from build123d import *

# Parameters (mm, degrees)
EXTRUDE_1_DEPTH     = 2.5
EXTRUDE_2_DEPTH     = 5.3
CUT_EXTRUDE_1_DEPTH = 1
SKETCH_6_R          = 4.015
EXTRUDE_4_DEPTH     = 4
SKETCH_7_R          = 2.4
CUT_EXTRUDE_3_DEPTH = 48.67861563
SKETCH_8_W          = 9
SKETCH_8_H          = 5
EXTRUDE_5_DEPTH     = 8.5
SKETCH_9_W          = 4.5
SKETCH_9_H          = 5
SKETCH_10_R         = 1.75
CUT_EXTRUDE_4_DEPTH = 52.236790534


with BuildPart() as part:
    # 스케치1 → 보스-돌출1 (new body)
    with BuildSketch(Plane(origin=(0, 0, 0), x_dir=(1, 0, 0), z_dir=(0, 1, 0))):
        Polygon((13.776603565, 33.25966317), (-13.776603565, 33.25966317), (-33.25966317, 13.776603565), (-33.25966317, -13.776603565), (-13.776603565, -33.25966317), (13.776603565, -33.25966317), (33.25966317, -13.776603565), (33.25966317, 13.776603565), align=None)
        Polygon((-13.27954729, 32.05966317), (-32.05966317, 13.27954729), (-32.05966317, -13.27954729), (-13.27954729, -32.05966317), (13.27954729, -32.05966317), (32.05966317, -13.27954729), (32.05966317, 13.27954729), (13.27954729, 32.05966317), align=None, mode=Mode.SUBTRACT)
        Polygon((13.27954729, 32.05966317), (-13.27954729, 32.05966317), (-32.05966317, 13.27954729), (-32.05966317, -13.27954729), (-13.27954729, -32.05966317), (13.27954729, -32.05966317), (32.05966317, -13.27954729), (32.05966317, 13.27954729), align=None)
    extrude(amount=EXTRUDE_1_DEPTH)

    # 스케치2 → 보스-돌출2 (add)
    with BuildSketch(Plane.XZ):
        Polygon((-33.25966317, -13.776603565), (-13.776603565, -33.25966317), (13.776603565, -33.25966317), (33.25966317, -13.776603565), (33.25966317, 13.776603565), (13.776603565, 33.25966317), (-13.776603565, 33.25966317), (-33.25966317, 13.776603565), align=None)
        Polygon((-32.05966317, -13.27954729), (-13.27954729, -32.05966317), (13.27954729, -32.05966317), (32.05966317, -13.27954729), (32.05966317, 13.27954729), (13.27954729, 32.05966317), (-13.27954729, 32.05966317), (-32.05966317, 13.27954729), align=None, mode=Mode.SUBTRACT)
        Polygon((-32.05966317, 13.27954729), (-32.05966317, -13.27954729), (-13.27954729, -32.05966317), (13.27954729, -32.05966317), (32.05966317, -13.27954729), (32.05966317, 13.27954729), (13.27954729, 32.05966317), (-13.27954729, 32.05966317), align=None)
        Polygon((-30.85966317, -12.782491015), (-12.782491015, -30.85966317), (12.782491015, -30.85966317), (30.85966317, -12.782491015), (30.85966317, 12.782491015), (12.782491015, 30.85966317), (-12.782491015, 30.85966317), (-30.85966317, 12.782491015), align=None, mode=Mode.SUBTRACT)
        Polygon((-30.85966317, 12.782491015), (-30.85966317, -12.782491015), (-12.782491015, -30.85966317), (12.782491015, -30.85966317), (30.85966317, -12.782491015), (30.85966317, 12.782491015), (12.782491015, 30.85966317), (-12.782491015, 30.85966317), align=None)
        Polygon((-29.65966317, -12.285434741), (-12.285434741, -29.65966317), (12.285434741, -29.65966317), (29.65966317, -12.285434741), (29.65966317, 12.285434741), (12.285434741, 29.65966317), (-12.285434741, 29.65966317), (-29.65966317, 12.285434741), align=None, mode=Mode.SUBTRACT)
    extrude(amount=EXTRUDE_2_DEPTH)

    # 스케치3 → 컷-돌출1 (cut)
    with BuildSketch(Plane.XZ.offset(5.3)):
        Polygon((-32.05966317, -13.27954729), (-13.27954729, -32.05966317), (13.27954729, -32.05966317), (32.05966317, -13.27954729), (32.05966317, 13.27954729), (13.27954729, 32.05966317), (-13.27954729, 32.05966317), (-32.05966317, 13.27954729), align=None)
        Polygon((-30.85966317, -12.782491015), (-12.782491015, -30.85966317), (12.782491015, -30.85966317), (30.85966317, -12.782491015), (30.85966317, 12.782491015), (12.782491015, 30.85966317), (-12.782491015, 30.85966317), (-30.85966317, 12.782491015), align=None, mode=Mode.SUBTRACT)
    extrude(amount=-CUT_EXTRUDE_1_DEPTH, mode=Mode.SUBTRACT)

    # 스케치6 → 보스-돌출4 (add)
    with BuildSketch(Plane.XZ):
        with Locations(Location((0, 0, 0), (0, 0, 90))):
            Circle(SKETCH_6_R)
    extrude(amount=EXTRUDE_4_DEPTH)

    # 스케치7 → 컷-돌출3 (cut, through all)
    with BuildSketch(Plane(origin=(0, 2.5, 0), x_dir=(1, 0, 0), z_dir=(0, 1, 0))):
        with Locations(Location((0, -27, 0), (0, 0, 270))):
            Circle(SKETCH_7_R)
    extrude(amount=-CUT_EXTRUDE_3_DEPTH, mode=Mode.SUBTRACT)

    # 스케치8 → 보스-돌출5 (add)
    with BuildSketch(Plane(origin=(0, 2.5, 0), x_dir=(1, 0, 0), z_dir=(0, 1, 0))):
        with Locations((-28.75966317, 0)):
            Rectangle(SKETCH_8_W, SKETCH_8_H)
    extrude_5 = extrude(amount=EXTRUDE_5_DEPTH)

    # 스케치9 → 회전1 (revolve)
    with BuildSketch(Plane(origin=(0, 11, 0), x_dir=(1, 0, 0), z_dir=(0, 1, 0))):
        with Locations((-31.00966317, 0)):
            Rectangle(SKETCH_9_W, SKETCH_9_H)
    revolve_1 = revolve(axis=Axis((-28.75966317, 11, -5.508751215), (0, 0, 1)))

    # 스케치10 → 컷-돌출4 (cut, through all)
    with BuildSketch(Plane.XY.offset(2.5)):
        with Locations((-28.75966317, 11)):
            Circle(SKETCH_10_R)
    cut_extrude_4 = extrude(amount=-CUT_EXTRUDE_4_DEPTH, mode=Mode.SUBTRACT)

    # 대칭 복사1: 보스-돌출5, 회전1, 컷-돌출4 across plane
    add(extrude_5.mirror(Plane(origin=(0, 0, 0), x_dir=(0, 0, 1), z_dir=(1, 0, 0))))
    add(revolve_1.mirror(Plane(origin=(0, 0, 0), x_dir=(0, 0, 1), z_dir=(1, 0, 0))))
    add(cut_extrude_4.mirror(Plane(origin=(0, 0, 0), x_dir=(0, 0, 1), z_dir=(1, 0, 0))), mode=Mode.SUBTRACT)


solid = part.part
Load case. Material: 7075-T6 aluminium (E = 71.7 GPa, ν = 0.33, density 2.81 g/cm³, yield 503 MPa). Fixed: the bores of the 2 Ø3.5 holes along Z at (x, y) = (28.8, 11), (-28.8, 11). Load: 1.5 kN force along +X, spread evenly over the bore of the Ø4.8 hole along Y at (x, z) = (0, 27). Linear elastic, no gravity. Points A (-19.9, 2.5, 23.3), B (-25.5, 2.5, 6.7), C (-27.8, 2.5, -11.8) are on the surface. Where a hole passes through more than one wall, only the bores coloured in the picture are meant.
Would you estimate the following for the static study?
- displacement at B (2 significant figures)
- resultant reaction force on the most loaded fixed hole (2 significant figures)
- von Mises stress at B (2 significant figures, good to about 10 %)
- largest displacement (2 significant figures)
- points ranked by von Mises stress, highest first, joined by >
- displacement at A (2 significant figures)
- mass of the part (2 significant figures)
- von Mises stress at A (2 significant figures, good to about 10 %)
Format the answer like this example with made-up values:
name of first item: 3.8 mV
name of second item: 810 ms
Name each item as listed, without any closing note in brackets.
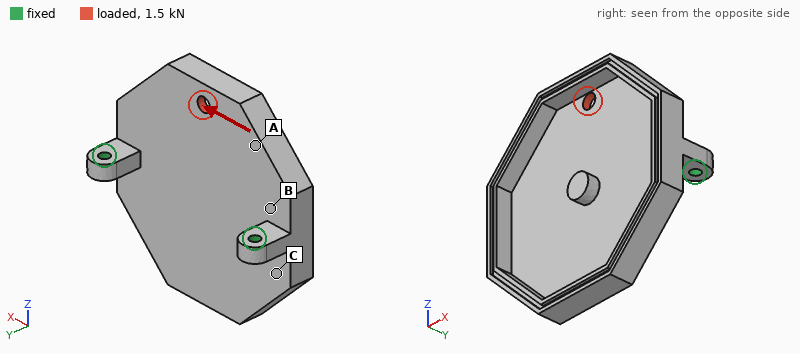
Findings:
displacement at B: 37 µm
resultant reaction force on the most loaded fixed hole: 1.0 kN
von Mises stress at B: 48 MPa
largest displacement: 69 µm
points ranked by von Mises stress, highest first, joined by >: B > A > C
displacement at A: 59 µm
mass of the part: 39 g
von Mises stress at A: 25 MPa
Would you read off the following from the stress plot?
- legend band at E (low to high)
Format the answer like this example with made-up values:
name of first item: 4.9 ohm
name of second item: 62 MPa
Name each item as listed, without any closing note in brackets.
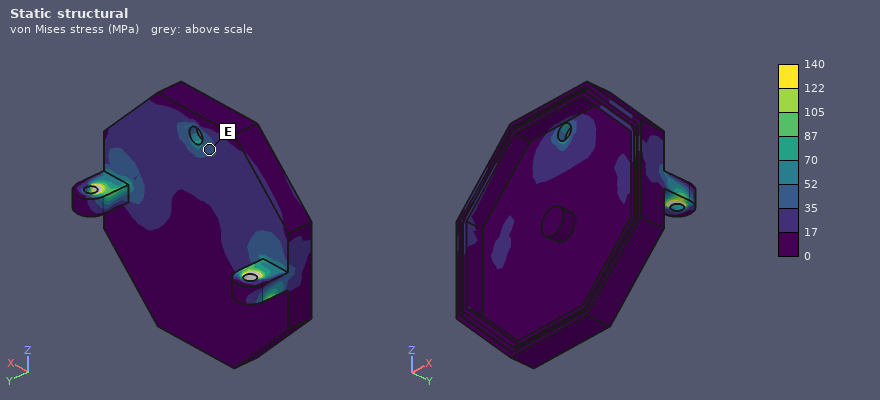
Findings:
legend band at E: 35 to 52 MPa
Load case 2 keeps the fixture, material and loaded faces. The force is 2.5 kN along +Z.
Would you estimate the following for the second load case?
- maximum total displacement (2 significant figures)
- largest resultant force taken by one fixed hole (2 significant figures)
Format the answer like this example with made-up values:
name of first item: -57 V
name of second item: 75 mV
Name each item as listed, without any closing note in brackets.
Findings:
maximum total displacement: 0.28 mm
largest resultant force taken by one fixed hole: 1.3 kN
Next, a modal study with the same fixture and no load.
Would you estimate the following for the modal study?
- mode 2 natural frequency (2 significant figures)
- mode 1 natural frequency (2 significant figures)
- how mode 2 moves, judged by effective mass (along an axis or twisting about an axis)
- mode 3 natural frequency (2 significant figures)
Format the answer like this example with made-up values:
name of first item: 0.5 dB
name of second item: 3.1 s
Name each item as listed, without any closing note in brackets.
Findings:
mode 2 natural frequency: 2700 Hz
mode 1 natural frequency: 1400 Hz
how mode 2 moves, judged by effective mass: along Y
mode 3 natural frequency: 4400 Hz
